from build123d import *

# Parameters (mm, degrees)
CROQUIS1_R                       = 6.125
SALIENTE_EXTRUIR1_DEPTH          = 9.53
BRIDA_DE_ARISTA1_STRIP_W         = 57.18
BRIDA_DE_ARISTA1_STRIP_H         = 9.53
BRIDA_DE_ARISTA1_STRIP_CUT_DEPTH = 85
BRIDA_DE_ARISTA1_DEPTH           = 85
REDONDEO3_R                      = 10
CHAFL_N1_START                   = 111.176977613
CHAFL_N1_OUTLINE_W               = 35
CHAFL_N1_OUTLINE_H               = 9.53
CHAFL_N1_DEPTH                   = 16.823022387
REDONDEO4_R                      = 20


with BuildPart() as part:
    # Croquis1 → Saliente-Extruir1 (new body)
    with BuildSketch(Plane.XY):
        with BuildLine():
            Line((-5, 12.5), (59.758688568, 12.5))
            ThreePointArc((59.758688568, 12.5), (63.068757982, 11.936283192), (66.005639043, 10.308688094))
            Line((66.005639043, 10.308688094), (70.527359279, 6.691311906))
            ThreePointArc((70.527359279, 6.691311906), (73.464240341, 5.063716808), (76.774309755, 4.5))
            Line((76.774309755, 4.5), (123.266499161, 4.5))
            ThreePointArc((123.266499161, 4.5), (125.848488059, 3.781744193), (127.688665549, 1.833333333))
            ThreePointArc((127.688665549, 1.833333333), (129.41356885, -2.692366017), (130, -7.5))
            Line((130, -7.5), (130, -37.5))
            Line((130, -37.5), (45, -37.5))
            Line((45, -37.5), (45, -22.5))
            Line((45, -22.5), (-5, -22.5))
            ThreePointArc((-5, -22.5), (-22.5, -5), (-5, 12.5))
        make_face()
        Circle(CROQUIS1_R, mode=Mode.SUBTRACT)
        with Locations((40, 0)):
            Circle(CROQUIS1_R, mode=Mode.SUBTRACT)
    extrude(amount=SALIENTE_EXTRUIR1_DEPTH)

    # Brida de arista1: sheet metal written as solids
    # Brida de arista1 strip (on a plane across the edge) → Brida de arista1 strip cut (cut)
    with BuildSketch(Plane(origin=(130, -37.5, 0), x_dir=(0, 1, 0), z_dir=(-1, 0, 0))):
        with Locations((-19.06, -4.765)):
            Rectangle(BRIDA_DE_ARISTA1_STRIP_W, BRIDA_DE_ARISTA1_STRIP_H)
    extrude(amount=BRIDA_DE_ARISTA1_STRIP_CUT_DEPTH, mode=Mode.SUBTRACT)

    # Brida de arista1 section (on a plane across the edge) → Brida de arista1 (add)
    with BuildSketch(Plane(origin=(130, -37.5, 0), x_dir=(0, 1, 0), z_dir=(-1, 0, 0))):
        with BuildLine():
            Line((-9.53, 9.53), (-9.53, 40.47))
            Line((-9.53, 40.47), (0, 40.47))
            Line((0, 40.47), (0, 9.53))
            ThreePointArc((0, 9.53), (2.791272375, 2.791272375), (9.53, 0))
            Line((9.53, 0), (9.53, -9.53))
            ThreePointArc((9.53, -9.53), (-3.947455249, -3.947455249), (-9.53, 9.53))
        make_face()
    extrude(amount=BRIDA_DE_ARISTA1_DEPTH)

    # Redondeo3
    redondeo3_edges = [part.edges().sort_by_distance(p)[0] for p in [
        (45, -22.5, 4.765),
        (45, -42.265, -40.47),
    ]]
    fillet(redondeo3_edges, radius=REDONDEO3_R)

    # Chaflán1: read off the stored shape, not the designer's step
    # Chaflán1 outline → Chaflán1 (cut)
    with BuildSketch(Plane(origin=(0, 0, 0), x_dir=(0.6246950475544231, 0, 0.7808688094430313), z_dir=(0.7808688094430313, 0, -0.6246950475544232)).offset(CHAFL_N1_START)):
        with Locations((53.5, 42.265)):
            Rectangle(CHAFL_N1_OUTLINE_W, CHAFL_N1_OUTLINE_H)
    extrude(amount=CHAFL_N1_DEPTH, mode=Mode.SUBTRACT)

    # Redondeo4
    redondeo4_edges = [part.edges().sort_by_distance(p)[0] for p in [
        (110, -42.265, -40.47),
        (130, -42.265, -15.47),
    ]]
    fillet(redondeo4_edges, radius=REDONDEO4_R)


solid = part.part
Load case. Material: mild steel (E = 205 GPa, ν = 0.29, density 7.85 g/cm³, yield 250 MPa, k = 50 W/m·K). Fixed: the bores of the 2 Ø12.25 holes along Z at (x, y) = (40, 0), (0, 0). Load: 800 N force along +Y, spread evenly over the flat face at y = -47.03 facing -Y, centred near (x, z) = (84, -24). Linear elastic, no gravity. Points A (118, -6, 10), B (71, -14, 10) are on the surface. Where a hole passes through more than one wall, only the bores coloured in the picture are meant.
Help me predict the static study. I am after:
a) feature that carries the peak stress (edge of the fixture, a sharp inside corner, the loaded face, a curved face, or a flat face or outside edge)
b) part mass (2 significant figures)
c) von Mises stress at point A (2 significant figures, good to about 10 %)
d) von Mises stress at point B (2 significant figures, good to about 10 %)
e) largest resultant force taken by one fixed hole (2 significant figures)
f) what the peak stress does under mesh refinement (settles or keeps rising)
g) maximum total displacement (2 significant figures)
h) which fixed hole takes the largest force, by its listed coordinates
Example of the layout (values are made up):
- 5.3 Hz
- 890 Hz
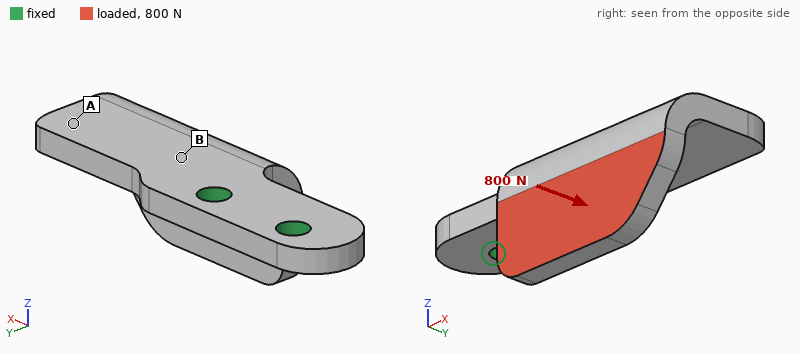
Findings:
- edge of the fixture
- 690 g
- 6.4 MPa
- 19 MPa
- 1.3 kN
- keeps rising
- 89 µm
- (40, 0)
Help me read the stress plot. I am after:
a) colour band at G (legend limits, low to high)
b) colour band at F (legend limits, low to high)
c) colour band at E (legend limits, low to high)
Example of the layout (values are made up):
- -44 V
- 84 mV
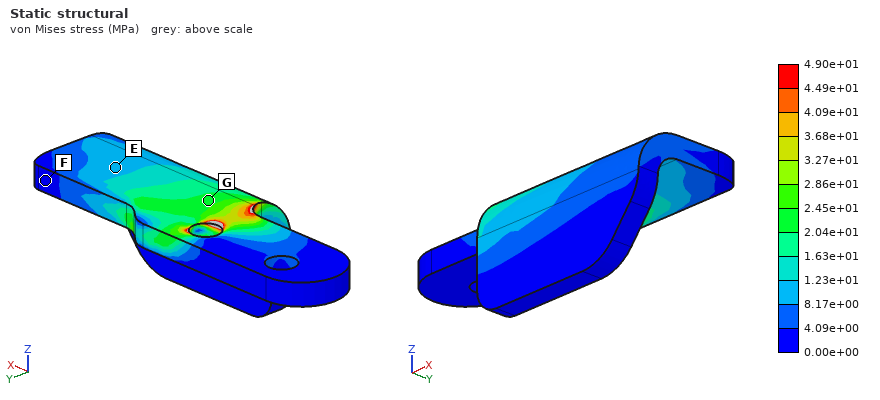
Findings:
- 2.04e+01 to 2.45e+01 MPa
- 0.00e+00 to 4.09e+00 MPa
- 8.17e+00 to 1.23e+01 MPa
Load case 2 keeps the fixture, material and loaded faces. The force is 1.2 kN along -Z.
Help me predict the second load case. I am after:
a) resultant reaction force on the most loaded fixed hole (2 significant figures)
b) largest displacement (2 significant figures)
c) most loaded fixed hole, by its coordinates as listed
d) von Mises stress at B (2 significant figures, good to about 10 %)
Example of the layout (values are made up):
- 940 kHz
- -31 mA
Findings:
- 1.5 kN
- 0.25 mm
- (40, 0)
- 45 MPa
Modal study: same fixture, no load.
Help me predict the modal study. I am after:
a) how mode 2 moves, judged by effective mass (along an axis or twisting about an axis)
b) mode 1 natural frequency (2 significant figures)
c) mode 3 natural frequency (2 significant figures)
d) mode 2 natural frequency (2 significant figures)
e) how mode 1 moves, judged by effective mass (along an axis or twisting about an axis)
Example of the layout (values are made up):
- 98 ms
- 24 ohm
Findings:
- along Y
- 650 Hz
- 2200 Hz
- 1300 Hz
- along Z
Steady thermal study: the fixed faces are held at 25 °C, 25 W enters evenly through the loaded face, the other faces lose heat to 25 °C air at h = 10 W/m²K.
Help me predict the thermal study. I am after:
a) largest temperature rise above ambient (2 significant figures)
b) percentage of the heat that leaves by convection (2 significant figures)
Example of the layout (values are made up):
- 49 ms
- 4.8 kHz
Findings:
- 59 K
- 24 %
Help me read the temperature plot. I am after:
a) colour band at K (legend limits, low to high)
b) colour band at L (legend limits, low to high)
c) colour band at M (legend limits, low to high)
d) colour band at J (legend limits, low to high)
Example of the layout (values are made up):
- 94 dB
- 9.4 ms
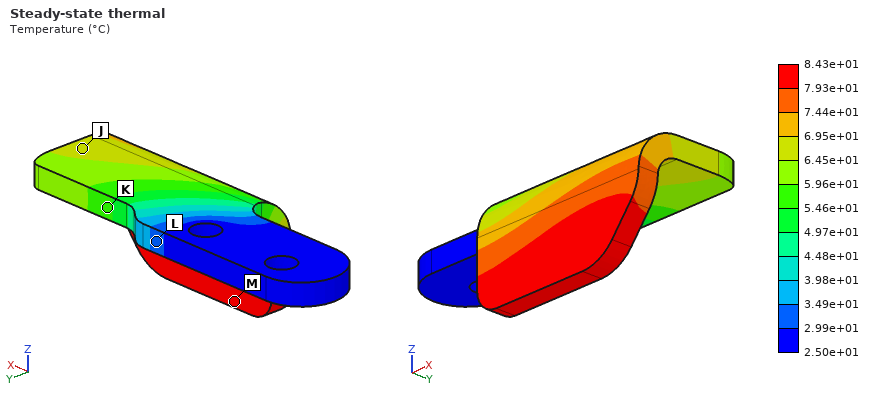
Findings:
- 5.46e+01 to 5.96e+01 °C
- 2.99e+01 to 3.49e+01 °C
- 7.93e+01 to 8.43e+01 °C
- 6.45e+01 to 6.95e+01 °C
